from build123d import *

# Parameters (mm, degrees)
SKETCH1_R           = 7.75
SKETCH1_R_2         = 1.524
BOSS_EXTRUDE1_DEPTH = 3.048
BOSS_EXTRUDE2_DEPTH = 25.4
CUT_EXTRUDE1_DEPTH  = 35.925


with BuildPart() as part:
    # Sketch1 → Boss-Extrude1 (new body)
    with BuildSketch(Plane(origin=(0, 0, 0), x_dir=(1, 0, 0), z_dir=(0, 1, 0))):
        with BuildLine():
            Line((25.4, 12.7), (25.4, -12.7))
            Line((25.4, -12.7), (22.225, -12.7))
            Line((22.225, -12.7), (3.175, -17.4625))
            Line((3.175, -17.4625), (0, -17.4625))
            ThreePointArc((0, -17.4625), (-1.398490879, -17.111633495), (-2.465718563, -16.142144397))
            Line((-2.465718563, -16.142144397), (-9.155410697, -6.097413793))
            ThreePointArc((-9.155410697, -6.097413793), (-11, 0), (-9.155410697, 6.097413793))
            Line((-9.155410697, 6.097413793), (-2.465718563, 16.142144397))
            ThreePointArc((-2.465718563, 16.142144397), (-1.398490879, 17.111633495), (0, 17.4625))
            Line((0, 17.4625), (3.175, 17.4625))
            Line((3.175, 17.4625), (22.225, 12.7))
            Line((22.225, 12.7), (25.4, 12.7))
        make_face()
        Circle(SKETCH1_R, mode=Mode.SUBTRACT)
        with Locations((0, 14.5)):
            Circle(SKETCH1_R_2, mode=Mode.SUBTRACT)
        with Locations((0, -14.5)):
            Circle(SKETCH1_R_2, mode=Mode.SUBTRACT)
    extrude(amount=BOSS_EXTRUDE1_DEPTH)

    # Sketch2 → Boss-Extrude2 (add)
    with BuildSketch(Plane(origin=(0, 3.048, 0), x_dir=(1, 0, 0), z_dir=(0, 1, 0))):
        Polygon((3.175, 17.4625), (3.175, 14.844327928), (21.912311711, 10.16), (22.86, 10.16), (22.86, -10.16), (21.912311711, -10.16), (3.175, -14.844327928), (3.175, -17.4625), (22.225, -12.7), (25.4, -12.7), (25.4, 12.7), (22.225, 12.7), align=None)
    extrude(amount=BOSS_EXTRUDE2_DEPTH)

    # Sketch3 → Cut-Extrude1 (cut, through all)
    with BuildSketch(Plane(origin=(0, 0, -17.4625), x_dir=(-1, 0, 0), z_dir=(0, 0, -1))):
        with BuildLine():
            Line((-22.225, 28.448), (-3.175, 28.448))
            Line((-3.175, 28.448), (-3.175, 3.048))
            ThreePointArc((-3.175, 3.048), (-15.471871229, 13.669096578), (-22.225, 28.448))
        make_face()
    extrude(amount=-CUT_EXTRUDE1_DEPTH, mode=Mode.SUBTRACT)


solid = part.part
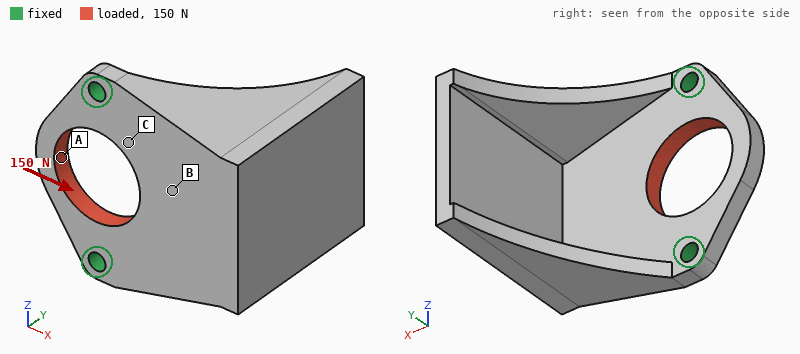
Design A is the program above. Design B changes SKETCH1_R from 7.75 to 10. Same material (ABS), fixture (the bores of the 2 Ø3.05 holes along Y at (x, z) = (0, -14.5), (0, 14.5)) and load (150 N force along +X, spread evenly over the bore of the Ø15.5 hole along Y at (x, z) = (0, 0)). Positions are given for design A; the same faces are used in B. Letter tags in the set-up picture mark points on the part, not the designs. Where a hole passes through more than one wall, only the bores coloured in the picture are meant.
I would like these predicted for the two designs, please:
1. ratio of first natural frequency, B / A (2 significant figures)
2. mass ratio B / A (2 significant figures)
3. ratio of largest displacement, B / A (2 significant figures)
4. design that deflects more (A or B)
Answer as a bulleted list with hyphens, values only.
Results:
- 0.94
- 0.92
- 2.5
- B
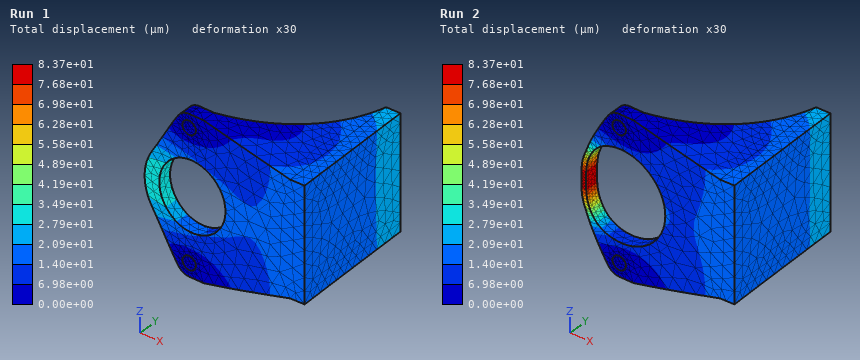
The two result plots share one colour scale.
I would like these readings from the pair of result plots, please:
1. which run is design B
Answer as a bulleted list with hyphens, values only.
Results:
- Run 2
